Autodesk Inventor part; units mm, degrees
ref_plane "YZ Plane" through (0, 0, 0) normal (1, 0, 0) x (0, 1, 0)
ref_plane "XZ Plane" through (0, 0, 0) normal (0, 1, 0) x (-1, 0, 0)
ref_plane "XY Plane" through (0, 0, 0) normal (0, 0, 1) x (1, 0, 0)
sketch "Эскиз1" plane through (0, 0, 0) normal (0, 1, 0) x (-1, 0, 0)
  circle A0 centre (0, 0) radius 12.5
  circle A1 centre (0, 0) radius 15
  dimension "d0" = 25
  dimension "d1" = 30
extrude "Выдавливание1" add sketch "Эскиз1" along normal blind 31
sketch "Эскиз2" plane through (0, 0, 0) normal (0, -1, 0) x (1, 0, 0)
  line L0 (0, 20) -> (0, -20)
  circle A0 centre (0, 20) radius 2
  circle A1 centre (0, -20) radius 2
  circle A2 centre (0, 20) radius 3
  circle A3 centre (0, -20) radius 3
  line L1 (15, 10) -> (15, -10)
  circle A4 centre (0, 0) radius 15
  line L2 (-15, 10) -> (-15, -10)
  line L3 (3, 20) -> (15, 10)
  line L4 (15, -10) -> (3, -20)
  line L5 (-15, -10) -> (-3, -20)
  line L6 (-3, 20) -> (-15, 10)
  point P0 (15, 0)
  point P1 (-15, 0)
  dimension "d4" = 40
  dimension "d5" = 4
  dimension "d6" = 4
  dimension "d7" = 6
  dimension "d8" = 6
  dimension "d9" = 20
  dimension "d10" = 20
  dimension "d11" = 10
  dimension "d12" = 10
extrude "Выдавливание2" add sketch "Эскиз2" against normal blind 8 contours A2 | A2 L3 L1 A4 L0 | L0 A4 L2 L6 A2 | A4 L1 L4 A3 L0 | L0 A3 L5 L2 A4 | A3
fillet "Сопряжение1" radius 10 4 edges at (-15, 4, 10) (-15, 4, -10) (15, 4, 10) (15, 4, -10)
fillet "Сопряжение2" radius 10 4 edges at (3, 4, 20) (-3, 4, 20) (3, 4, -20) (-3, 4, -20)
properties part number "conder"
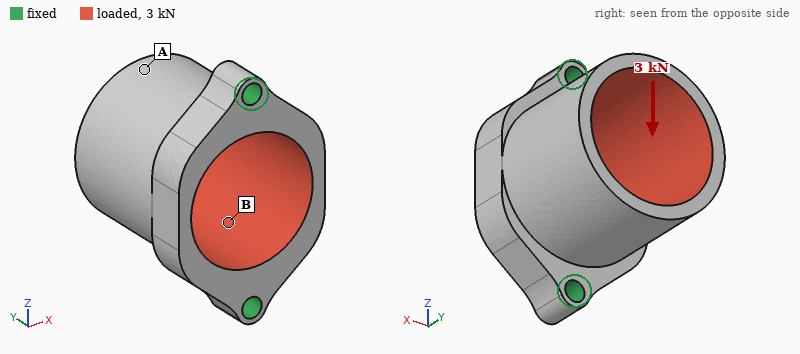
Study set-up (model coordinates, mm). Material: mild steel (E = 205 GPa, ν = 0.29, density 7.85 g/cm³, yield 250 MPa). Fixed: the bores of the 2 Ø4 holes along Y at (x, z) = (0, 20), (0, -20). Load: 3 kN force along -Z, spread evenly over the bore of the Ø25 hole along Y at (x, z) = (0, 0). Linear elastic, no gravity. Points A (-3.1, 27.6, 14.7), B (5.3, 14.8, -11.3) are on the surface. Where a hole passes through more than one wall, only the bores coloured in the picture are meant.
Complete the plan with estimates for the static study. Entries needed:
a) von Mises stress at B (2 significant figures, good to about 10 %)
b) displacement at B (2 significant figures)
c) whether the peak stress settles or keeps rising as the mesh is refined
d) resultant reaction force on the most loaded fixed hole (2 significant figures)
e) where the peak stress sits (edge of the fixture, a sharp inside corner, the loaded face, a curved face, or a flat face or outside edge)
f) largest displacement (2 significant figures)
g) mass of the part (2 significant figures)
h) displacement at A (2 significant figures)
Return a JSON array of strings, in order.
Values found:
["29 MPa", "4.4 µm", "keeps rising", "1.8 kN", "edge of the fixture", "9.0 µm", "68 g", "8.3 µm"]
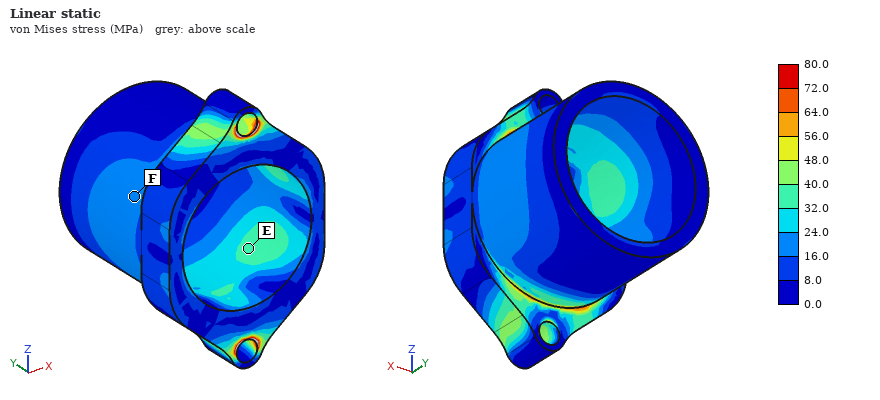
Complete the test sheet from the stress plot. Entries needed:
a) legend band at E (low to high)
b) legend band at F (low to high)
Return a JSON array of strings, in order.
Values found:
["32.0 to 40.0 MPa", "16.0 to 24.0 MPa"]
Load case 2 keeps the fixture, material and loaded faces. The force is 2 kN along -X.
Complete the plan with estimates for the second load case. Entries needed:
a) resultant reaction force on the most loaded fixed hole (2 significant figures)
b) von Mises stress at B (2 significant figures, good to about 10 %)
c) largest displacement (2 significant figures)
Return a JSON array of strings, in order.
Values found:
["1.0 kN", "24 MPa", "30 µm"]
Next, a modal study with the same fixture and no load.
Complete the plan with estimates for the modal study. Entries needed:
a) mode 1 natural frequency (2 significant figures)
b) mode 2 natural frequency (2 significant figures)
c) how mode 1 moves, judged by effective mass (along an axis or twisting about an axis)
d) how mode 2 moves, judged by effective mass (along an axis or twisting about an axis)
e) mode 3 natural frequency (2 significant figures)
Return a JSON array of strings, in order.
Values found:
["6100 Hz", "10 kHz", "along X", "along Y", "11 kHz"]
